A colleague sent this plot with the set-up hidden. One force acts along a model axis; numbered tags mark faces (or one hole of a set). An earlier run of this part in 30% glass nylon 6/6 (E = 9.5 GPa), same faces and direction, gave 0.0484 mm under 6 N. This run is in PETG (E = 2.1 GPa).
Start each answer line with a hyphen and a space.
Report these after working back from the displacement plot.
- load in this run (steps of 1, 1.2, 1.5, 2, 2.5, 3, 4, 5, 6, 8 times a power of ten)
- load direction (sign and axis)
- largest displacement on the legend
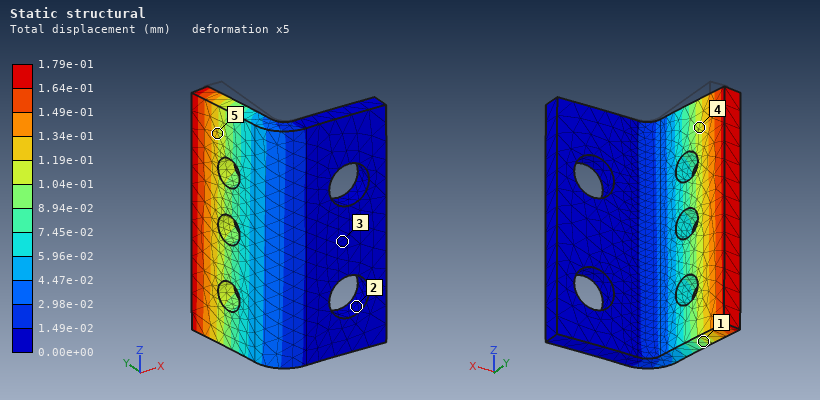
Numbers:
- 5 N
- -X
- 1.79e-01 mm
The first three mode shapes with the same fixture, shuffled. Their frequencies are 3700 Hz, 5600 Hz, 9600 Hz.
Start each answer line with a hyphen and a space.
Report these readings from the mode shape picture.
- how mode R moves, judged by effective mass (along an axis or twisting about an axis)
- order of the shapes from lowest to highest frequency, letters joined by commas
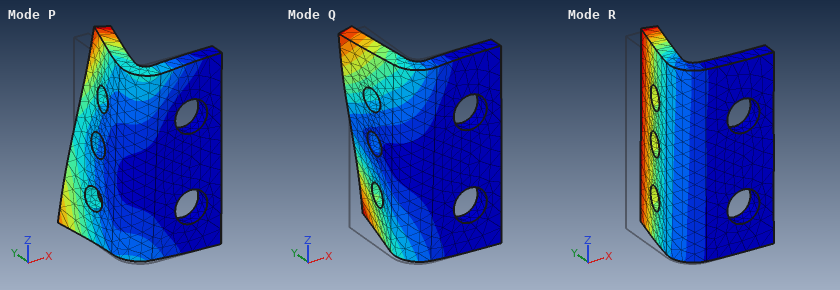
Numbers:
- along X
- R, Q, P
